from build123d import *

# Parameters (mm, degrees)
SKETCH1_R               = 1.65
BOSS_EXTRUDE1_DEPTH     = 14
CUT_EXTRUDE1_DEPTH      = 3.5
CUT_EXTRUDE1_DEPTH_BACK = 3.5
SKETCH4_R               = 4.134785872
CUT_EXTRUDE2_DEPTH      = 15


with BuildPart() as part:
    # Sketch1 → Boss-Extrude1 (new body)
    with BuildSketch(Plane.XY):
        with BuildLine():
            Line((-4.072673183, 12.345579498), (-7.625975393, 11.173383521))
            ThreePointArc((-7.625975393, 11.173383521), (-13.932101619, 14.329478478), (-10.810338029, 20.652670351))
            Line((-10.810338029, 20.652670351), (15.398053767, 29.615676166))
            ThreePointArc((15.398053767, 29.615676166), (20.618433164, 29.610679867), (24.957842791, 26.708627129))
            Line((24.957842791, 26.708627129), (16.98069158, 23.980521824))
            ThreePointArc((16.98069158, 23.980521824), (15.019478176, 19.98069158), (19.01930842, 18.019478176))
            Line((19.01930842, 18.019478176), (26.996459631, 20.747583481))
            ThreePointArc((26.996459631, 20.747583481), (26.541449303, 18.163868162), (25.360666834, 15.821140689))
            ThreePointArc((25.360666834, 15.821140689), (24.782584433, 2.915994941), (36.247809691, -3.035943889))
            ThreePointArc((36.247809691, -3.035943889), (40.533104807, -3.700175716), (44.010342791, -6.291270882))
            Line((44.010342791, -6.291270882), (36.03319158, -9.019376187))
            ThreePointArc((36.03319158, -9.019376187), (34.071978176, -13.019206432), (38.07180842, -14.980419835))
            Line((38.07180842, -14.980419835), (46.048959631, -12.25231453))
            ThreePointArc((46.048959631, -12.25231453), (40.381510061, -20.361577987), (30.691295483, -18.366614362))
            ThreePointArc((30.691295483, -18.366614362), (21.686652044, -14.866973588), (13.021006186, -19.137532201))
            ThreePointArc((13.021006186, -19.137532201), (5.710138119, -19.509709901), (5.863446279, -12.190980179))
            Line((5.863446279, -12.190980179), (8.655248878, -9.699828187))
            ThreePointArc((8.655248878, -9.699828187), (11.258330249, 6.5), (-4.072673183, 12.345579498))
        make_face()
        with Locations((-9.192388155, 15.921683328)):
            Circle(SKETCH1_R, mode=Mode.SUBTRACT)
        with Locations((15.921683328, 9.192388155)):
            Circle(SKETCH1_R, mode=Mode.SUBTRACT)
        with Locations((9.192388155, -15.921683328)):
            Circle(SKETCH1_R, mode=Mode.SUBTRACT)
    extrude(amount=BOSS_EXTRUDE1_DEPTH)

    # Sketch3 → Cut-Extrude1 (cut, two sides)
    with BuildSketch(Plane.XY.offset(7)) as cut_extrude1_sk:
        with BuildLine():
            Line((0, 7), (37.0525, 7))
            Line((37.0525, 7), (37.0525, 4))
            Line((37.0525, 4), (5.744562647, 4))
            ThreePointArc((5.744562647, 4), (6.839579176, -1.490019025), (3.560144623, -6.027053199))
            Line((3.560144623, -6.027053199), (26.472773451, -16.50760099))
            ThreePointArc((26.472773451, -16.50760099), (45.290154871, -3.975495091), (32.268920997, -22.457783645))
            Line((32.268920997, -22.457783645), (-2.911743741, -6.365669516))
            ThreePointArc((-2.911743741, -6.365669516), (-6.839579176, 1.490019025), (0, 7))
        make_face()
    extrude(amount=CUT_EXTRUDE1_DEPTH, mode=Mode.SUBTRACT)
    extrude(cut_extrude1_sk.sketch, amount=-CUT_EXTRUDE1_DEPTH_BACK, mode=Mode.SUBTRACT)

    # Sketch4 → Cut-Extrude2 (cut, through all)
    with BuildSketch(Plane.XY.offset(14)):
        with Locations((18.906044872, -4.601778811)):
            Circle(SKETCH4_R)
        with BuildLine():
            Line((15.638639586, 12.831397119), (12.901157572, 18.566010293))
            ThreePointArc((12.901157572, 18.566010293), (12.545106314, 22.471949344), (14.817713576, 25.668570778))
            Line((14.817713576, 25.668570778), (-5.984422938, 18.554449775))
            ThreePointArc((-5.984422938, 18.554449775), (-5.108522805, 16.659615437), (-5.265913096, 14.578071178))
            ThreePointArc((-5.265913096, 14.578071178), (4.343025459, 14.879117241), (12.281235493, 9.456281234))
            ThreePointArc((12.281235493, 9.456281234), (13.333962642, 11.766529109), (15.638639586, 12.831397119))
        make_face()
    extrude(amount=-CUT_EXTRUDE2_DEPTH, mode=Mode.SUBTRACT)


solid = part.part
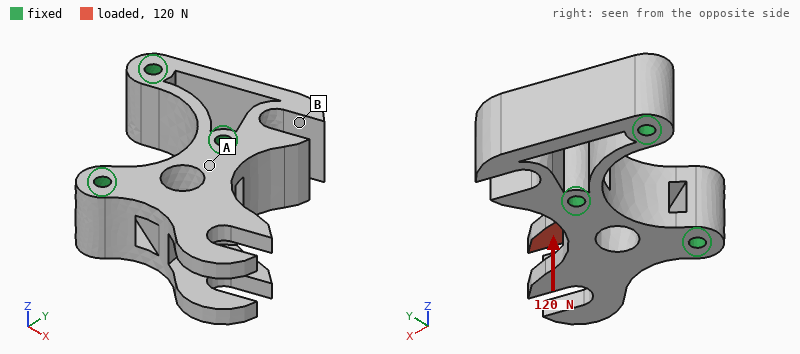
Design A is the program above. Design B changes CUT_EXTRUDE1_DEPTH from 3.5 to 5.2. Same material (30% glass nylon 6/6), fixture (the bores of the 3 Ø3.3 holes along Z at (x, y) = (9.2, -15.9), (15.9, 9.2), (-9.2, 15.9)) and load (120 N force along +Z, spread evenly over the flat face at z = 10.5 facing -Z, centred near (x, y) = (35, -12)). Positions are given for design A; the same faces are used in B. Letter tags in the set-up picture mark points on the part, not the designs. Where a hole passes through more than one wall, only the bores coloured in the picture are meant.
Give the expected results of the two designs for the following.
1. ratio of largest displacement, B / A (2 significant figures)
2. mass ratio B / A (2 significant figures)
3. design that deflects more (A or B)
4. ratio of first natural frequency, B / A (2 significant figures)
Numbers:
5.3
0.95
B
0.64
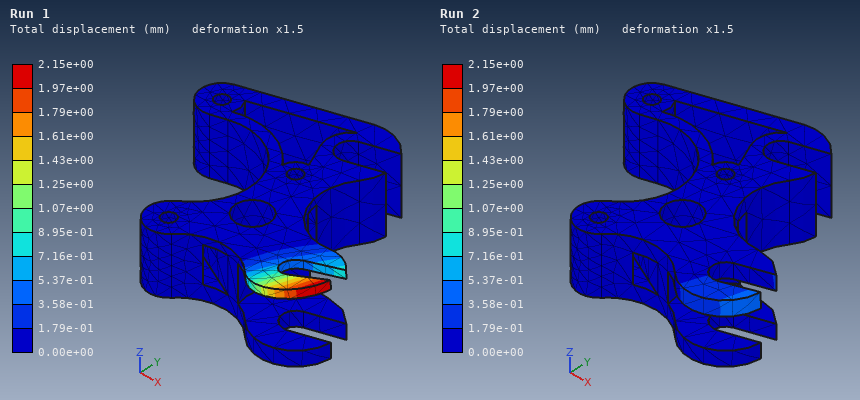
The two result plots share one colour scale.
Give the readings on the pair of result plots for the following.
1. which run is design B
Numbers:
Run 1
